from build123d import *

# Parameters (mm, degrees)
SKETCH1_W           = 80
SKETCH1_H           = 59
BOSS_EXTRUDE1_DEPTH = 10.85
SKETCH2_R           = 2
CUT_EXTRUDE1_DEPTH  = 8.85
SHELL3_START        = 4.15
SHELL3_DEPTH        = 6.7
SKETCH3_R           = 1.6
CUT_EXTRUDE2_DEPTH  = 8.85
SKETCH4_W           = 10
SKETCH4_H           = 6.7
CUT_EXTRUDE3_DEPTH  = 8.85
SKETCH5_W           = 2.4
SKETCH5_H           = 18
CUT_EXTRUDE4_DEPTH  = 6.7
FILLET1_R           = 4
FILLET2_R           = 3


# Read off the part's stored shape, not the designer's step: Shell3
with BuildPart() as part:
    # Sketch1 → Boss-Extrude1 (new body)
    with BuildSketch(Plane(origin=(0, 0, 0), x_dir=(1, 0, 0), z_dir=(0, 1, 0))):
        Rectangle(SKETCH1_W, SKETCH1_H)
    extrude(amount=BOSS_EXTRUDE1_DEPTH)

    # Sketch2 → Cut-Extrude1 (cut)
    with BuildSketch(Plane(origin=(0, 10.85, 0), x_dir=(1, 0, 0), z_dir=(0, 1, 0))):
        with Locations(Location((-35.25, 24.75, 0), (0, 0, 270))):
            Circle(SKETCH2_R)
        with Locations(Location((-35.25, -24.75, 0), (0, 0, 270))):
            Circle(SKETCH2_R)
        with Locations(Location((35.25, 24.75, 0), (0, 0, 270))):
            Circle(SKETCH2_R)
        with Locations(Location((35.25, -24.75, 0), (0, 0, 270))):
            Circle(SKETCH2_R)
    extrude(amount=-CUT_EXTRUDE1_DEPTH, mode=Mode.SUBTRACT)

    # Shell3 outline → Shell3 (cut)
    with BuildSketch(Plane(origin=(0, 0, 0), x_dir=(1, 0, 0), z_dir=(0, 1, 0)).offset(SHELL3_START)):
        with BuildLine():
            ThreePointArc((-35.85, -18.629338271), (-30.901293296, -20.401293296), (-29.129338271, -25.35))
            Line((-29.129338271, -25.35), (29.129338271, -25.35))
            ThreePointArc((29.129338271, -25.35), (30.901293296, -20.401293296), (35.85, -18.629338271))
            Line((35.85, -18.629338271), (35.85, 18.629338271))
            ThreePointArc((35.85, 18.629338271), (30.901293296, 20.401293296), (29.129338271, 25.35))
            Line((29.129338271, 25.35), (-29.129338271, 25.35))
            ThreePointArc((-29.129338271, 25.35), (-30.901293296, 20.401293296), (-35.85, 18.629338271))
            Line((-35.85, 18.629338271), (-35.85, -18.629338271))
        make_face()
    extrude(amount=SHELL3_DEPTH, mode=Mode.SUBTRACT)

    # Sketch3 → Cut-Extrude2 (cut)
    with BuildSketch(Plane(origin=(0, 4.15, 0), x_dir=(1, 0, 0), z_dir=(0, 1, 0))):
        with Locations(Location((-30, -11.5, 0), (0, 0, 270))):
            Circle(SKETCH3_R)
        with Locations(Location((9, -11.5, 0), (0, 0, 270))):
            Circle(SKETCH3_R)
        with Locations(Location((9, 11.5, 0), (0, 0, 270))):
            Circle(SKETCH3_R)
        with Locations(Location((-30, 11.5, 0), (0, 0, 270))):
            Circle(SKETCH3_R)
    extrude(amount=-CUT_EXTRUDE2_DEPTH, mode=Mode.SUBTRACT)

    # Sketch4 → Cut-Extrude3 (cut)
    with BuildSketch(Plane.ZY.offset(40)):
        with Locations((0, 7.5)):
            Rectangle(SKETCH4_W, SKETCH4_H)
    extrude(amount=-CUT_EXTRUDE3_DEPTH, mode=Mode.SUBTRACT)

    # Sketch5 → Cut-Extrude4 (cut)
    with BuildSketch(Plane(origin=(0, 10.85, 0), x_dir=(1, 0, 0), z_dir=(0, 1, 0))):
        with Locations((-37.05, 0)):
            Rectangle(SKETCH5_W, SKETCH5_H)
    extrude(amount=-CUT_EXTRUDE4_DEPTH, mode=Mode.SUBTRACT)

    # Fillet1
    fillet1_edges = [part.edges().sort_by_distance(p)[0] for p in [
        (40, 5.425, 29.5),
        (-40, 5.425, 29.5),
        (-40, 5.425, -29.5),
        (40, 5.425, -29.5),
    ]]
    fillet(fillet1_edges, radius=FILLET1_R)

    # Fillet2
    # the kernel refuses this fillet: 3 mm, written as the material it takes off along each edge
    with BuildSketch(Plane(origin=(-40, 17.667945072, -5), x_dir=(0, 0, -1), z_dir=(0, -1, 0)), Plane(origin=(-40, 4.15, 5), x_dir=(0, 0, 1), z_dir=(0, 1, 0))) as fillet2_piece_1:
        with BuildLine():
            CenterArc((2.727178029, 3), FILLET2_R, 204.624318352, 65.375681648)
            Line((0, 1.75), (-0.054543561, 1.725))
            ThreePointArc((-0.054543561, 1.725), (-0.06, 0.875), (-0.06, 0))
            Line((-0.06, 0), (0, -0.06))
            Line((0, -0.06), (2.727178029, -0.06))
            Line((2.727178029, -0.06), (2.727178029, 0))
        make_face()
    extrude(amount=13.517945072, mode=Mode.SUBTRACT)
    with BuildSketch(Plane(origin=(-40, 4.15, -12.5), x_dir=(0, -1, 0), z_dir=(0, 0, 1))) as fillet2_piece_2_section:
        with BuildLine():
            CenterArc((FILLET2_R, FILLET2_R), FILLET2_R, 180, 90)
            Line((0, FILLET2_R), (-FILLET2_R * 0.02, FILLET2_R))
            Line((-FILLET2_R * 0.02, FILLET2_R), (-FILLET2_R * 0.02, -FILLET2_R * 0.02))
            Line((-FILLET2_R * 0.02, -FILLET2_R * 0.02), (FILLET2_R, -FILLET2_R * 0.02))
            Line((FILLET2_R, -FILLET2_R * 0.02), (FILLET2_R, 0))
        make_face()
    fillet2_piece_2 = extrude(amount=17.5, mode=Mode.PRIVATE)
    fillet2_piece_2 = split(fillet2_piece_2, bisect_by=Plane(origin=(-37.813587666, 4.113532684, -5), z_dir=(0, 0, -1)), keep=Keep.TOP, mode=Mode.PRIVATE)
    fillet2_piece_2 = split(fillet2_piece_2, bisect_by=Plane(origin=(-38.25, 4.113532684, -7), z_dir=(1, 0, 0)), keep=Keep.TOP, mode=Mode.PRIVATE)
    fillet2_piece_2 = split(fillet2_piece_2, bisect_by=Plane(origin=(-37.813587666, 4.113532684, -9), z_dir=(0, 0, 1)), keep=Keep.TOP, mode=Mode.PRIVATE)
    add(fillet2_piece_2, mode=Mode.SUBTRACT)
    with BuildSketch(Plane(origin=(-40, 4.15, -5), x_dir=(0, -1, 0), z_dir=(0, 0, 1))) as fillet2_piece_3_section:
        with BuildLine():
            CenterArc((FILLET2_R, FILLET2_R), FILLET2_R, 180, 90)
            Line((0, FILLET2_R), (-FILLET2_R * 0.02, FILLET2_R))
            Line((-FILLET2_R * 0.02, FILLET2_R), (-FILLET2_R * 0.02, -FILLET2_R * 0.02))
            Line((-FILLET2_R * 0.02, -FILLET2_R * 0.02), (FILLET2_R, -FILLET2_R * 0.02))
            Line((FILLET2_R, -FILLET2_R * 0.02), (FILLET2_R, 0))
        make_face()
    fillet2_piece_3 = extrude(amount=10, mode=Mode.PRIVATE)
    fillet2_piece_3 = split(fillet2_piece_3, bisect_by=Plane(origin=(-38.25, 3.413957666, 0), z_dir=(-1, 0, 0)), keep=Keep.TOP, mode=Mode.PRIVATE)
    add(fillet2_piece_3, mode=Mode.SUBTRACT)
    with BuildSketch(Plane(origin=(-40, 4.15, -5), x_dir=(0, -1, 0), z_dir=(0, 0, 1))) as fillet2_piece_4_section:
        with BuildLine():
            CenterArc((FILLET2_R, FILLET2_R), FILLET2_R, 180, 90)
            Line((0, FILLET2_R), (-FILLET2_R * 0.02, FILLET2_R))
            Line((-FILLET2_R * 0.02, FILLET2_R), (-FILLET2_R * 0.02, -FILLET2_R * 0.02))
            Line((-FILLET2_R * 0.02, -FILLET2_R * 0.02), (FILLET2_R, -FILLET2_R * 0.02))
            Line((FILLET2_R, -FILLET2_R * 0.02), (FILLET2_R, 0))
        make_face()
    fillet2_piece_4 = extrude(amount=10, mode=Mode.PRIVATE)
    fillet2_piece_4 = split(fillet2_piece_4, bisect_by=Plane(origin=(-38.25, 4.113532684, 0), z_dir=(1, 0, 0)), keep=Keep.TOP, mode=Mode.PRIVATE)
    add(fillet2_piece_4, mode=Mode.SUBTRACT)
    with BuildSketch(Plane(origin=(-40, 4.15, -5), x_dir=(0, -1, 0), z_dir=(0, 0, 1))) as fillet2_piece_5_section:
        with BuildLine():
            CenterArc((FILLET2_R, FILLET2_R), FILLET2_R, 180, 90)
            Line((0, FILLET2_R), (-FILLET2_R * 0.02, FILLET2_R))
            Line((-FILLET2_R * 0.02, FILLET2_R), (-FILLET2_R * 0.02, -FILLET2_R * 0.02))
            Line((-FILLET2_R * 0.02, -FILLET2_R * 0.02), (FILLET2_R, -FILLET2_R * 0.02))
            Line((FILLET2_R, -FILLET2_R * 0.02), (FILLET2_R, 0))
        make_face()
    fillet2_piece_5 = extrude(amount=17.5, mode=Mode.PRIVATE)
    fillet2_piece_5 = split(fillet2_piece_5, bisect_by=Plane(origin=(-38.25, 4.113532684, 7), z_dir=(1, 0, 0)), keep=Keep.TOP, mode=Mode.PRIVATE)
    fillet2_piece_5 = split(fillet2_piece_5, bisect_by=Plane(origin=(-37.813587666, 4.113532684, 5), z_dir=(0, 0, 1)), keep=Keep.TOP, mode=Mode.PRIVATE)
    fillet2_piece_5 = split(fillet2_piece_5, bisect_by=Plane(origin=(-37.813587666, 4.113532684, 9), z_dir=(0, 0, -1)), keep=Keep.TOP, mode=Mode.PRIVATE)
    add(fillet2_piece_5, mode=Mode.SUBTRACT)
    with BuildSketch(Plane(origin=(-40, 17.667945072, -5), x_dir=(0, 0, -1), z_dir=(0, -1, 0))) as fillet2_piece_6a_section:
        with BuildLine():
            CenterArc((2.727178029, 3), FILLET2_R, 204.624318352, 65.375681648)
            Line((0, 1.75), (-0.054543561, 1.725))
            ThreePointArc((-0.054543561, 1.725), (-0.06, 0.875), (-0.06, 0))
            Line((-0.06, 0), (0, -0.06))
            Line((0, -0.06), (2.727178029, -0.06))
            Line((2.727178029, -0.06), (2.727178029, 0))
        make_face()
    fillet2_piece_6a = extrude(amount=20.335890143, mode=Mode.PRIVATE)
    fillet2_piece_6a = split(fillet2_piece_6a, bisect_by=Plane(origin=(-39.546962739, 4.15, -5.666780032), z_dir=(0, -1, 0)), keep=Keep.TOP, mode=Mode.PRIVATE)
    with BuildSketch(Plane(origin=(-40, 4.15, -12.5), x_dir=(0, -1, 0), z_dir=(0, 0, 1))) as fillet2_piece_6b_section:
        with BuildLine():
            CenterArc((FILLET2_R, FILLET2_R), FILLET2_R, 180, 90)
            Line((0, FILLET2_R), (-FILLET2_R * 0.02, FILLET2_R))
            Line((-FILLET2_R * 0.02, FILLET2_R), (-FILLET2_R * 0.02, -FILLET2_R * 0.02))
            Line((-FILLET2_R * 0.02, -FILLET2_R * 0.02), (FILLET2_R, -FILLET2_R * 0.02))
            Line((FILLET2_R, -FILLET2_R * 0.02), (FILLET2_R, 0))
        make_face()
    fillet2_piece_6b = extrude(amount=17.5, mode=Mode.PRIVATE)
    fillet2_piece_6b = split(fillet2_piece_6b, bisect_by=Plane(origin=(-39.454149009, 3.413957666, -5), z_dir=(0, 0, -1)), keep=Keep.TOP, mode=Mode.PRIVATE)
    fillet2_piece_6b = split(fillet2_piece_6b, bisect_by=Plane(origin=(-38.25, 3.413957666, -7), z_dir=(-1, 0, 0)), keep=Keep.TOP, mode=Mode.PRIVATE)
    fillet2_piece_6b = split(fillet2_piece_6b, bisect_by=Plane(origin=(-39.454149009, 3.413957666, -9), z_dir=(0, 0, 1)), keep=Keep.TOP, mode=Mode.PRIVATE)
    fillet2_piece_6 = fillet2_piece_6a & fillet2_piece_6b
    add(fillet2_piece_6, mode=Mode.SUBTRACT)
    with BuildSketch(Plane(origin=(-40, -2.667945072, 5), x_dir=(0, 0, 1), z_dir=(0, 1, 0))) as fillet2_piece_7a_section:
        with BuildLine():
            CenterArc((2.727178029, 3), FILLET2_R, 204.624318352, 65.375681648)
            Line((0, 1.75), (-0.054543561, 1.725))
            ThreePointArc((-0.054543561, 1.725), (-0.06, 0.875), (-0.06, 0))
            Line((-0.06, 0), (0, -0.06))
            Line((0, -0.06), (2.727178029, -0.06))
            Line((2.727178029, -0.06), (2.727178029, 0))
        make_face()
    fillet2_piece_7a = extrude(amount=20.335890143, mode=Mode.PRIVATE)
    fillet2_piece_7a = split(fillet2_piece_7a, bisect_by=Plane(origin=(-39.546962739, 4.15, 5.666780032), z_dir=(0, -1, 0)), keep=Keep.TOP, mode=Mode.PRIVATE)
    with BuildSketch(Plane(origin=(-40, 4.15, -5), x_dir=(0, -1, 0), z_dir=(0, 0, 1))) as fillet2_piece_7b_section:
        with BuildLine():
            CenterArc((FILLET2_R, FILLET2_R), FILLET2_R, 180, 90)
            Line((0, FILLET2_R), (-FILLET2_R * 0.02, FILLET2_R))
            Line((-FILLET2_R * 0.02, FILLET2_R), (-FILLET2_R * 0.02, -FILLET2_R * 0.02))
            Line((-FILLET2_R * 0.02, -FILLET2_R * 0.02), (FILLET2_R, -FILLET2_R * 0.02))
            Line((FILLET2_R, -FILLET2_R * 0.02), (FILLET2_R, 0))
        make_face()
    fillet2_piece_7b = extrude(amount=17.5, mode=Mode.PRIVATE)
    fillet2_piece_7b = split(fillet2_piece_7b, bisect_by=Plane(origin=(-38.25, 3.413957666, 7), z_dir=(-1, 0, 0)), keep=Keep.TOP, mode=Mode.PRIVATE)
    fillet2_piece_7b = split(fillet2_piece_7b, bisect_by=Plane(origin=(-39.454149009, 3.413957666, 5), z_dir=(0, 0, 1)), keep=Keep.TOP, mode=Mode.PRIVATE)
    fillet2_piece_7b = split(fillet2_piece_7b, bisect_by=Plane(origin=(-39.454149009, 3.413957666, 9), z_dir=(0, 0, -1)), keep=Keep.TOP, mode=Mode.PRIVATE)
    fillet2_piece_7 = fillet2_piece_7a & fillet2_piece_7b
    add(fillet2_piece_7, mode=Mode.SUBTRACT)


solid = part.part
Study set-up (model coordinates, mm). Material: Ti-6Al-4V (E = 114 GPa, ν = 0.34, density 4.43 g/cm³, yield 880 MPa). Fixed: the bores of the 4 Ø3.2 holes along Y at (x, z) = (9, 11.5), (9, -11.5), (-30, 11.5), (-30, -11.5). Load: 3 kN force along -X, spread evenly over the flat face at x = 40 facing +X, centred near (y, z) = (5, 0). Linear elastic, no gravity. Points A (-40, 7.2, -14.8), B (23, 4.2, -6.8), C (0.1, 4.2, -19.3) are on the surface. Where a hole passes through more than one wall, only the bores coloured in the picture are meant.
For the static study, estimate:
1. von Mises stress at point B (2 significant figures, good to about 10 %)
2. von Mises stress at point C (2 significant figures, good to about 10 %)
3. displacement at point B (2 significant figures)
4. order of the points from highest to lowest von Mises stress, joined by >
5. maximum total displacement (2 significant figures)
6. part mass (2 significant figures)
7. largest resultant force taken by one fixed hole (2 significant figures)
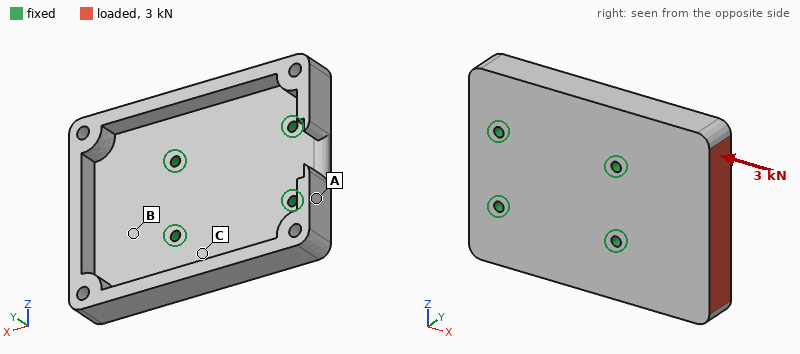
33 MPa
11 MPa
11 µm
B > C > A
55 µm
120 g
1.2 kN
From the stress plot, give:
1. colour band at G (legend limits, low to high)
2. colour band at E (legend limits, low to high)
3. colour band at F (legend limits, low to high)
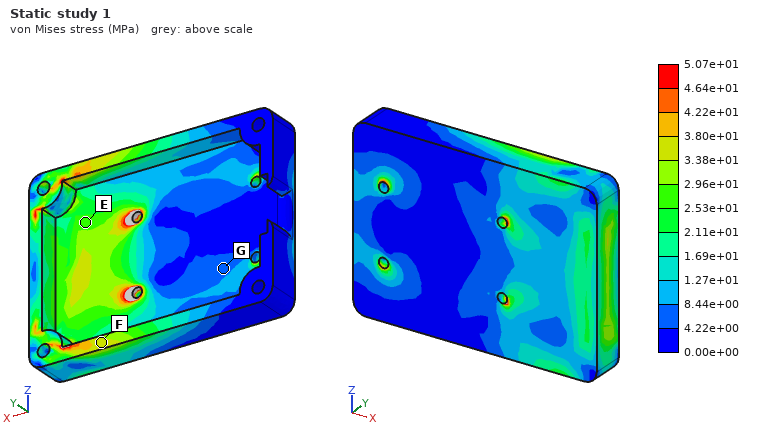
4.22e+00 to 8.44e+00 MPa
2.53e+01 to 2.96e+01 MPa
3.38e+01 to 3.80e+01 MPa
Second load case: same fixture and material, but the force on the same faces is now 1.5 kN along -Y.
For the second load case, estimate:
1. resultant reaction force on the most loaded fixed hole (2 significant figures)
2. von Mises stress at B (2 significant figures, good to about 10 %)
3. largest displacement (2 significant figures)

1.3 kN
48 MPa
0.20 mm
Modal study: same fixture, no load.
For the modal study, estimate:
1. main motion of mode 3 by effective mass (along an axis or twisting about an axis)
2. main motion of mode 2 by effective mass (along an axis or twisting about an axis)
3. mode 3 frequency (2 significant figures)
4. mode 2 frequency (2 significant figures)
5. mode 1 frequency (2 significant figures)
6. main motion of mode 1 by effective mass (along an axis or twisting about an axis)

along Y
twisting about X
6400 Hz
3900 Hz
3300 Hz
along Y
